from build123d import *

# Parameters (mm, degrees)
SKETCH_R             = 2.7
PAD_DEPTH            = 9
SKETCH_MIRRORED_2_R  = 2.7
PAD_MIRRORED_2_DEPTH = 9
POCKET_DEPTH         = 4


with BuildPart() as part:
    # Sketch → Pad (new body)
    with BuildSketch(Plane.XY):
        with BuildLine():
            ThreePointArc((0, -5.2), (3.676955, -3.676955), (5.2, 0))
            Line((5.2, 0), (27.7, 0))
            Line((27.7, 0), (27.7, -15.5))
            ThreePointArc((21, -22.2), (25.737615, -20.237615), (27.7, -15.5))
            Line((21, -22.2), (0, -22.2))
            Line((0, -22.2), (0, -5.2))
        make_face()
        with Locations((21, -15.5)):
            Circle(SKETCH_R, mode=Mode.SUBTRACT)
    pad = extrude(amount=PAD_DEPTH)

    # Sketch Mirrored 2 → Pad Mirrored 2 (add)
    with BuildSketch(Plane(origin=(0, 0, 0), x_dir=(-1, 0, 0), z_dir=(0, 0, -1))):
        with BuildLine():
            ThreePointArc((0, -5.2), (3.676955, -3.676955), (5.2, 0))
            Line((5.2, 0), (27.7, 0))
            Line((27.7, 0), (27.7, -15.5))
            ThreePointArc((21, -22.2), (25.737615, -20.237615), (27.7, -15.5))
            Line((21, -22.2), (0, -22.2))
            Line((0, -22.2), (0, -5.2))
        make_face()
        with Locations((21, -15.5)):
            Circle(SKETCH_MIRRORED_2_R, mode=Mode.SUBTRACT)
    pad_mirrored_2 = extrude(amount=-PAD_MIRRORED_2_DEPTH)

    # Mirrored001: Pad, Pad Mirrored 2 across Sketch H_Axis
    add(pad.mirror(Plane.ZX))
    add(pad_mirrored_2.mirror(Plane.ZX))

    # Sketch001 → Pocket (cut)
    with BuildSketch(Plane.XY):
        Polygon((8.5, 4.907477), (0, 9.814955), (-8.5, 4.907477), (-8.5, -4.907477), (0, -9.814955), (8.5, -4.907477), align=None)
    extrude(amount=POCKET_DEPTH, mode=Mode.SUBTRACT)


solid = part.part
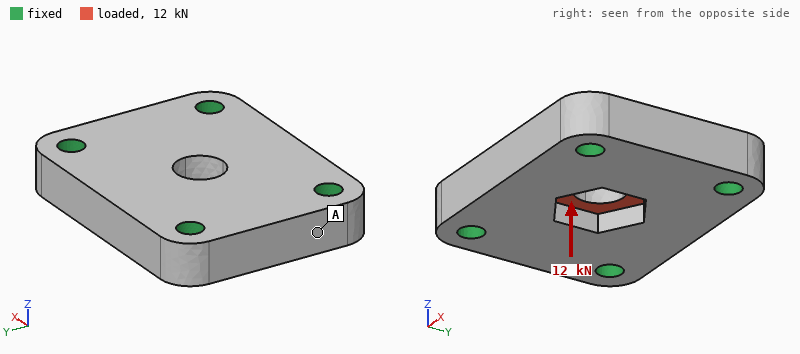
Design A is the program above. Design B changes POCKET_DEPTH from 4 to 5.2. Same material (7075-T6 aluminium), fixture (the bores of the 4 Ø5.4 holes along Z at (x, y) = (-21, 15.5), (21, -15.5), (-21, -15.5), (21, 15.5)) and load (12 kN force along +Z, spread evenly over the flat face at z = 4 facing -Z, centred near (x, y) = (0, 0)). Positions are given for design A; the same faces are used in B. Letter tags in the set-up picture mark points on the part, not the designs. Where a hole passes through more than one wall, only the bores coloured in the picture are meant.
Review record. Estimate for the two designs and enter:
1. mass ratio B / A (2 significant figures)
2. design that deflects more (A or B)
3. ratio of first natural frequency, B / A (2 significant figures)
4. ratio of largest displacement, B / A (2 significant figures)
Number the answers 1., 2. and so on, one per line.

1. 0.99
2. B
3. 1.0
4. 1.1
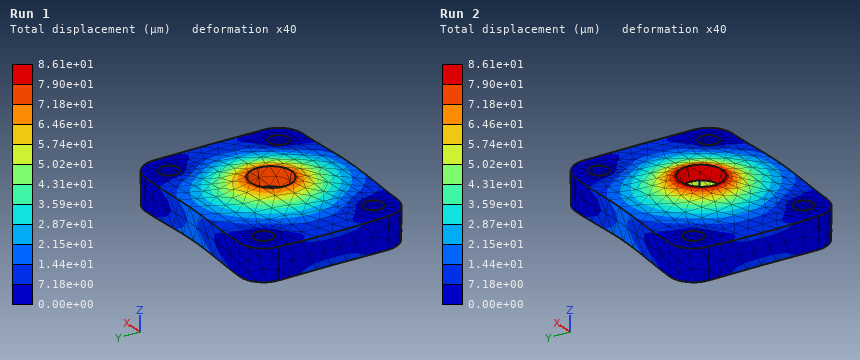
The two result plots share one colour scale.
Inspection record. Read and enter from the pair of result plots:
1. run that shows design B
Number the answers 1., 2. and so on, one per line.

1. Run 2
